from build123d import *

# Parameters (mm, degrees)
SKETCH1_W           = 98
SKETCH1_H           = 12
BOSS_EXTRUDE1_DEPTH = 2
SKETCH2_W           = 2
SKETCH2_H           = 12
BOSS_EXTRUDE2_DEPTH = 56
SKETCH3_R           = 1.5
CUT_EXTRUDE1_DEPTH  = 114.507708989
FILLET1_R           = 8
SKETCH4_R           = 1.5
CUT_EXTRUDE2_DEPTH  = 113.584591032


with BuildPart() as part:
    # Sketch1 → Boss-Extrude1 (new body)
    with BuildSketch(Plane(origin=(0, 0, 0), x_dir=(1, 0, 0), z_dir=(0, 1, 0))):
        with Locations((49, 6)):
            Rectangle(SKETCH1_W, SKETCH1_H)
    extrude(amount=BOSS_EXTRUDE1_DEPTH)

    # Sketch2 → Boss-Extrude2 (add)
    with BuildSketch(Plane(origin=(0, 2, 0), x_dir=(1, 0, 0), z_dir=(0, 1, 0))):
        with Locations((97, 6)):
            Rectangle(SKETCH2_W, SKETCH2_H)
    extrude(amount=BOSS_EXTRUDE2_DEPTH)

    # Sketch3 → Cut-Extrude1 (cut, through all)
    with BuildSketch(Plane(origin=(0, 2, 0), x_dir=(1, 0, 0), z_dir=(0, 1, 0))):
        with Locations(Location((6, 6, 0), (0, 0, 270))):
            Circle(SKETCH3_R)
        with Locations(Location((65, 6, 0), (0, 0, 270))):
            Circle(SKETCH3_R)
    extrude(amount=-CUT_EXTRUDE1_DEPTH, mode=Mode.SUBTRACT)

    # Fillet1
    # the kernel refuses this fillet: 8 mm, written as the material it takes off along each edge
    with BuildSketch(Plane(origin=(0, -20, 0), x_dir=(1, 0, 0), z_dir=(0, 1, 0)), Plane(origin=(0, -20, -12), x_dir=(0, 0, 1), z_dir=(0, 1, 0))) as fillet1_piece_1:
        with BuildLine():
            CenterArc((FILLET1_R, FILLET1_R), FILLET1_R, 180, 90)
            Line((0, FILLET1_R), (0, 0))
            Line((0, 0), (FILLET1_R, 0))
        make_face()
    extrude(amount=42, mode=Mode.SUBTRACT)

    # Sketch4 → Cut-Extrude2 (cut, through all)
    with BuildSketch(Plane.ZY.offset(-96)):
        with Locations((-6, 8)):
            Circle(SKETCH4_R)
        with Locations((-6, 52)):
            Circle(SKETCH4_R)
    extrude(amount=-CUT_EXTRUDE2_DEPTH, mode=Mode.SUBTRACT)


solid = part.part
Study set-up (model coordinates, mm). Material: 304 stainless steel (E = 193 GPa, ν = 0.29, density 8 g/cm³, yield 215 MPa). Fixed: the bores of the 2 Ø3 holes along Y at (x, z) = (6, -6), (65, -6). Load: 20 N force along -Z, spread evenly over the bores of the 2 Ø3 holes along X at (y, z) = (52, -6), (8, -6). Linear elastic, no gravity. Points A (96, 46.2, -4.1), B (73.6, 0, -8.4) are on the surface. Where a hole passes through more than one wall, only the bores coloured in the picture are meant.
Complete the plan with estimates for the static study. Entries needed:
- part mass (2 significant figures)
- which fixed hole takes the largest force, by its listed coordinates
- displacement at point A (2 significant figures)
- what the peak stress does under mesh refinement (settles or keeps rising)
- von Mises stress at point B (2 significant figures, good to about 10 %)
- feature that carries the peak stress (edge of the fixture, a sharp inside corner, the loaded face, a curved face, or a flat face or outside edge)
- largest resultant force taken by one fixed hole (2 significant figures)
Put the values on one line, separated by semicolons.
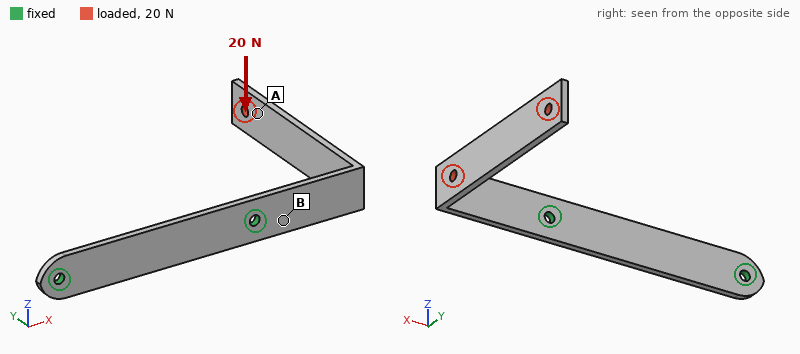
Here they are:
29 g; (65, -6); 0.37 mm; keeps rising; 65 MPa; edge of the fixture; 25 N
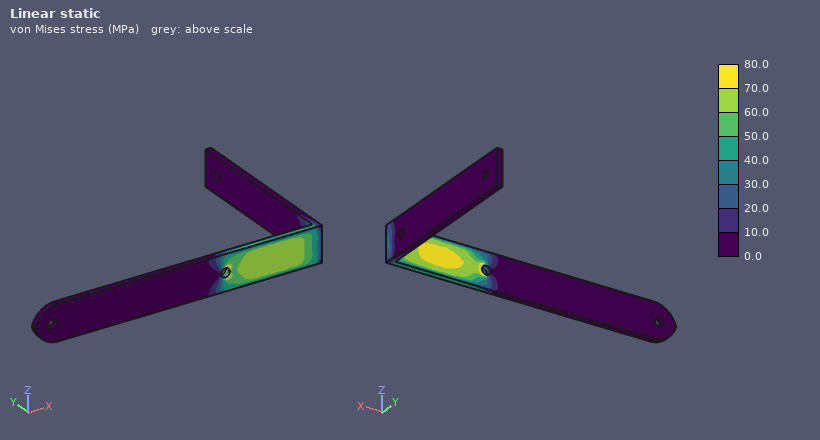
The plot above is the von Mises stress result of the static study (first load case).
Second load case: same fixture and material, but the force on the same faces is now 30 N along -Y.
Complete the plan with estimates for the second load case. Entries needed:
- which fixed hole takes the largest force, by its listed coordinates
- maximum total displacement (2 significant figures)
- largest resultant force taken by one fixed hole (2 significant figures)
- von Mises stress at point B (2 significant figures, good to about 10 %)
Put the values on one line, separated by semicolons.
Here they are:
(65, -6); 0.58 mm; 30 N; 84 MPa
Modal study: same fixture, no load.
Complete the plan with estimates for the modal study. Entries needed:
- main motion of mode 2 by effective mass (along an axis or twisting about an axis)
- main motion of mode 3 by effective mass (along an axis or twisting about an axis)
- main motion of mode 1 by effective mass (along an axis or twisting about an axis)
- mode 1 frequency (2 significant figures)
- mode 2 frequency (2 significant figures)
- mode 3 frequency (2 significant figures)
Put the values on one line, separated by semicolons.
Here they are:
along Z; along Y; along X; 260 Hz; 390 Hz; 840 Hz
